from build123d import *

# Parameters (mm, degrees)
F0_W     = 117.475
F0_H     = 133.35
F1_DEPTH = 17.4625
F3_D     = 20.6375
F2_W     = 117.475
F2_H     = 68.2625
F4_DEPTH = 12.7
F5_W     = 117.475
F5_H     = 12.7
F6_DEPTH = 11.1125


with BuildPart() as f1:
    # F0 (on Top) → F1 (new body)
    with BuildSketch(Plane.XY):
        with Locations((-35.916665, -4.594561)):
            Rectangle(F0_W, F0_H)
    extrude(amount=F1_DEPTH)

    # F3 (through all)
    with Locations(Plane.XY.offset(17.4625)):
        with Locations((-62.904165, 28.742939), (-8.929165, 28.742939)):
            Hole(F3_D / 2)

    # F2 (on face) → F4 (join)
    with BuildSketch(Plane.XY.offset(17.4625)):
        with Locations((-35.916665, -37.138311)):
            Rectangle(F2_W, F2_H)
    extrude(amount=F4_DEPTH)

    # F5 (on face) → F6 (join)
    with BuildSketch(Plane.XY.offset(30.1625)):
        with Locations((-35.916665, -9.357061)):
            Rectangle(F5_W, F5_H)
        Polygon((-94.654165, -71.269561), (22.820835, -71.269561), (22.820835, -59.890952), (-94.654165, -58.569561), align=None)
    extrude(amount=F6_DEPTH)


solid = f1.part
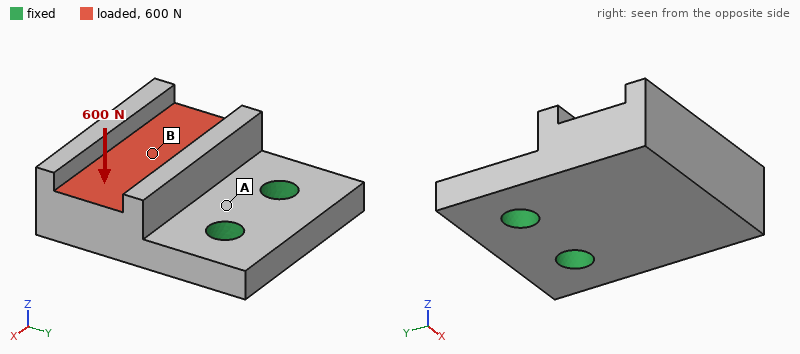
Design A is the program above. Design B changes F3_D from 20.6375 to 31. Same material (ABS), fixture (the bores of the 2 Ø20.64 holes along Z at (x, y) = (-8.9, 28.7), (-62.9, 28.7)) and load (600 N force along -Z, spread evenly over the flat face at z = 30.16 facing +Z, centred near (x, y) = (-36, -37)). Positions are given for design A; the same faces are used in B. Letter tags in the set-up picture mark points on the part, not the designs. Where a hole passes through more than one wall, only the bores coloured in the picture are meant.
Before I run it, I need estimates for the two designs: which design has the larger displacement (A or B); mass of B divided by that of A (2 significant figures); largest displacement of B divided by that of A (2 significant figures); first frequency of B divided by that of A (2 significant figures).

A
0.96
0.74
1.2
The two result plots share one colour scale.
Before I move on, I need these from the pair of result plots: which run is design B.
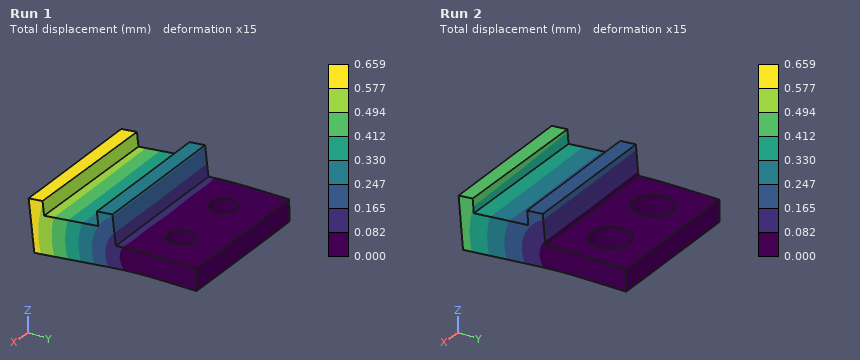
Run 2
